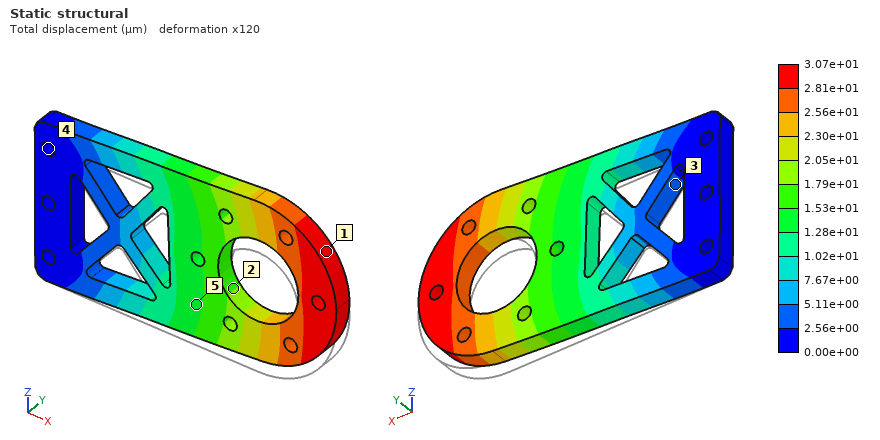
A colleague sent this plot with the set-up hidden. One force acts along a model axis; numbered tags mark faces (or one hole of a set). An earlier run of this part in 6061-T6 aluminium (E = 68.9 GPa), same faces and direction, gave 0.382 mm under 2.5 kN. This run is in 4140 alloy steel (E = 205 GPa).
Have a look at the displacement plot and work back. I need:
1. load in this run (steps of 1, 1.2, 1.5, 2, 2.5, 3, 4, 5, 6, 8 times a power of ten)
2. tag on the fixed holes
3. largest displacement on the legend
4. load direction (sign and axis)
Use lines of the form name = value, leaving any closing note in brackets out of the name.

load in this run = 600 N
tag on the fixed holes = 4
largest displacement on the legend = 3.07e+01 µm
load direction = +Z
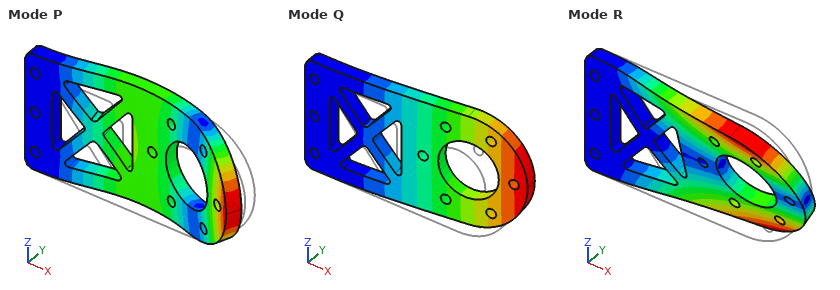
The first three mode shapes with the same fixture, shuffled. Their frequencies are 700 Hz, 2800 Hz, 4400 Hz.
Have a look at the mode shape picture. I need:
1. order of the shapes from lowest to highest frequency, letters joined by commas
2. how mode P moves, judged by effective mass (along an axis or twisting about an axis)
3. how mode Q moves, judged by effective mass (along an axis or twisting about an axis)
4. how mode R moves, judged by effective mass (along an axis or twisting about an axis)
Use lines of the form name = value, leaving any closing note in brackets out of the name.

order of the shapes from lowest to highest frequency, letters joined by commas = Q, R, P
how mode P moves, judged by effective mass = along Y
how mode Q moves, judged by effective mass = along Y
how mode R moves, judged by effective mass = twisting about X
